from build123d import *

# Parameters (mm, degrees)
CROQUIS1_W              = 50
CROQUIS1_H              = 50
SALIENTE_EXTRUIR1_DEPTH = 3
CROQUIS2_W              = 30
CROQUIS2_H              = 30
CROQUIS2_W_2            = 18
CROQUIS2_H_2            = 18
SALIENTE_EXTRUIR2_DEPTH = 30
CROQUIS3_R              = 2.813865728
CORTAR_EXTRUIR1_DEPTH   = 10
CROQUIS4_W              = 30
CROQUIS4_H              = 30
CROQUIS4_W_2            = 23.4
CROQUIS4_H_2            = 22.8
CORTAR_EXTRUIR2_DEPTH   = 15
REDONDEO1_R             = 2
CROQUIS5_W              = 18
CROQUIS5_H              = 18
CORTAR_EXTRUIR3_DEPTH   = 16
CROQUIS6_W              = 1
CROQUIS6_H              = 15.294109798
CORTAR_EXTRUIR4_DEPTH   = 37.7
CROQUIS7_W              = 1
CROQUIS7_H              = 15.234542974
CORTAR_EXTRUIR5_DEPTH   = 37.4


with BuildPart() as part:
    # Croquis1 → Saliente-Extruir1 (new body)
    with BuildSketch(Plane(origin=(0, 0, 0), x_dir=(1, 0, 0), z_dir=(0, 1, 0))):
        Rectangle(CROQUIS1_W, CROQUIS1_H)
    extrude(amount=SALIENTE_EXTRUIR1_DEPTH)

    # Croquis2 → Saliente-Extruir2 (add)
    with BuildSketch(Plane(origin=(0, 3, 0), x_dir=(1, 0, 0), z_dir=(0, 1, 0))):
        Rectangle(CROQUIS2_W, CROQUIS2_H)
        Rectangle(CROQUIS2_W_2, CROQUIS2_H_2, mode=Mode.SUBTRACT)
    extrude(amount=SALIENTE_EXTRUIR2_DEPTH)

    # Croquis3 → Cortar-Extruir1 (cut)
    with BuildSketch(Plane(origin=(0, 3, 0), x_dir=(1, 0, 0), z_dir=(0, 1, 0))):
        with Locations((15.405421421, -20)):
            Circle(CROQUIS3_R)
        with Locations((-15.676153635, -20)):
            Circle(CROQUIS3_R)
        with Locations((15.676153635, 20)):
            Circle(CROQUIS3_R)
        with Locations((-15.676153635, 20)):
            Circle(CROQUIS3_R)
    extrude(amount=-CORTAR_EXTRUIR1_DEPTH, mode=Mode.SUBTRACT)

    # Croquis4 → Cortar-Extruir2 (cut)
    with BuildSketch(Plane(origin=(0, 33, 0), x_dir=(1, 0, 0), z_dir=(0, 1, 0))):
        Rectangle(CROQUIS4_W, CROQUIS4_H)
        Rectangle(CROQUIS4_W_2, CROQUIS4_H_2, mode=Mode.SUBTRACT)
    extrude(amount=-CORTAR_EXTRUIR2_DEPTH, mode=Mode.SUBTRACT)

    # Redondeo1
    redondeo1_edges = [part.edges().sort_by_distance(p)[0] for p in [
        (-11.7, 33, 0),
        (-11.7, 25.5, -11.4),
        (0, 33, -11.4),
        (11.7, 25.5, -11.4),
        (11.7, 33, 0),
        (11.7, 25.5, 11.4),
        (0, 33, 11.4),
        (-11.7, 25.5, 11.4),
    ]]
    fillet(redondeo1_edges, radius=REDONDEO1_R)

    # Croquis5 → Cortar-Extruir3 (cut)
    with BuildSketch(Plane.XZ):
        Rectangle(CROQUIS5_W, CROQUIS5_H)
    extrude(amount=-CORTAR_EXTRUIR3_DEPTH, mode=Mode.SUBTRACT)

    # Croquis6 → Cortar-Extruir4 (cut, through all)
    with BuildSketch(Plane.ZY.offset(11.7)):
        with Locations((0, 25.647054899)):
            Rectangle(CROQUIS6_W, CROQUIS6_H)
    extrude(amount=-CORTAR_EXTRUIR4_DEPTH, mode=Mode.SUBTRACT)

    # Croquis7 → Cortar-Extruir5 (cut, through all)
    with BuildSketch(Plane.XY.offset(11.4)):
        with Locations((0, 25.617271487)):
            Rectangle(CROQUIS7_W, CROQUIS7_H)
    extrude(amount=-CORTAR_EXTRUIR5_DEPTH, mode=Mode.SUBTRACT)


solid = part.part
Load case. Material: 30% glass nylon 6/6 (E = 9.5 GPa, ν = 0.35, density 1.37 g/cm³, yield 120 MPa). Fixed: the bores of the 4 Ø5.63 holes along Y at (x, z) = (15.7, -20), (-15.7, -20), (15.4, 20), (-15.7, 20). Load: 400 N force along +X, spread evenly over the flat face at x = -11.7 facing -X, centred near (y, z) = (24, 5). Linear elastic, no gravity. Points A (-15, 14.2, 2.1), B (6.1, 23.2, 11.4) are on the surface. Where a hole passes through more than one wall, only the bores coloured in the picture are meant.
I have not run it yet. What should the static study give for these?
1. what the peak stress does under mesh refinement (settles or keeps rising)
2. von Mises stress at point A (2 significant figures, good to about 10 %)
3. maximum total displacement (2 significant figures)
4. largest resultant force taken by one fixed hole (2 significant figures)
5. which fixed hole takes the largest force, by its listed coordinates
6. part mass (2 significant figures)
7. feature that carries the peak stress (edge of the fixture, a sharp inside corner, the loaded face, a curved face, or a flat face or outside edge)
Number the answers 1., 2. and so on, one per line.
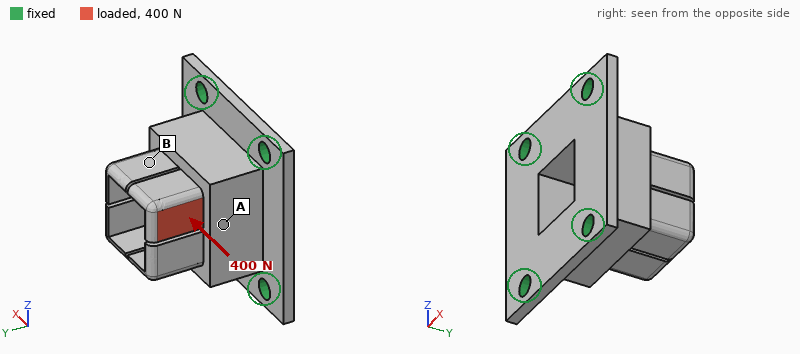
1. keeps rising
2. 16 MPa
3. 0.48 mm
4. 280 N
5. (15.4, 20)
6. 24 g
7. a sharp inside corner
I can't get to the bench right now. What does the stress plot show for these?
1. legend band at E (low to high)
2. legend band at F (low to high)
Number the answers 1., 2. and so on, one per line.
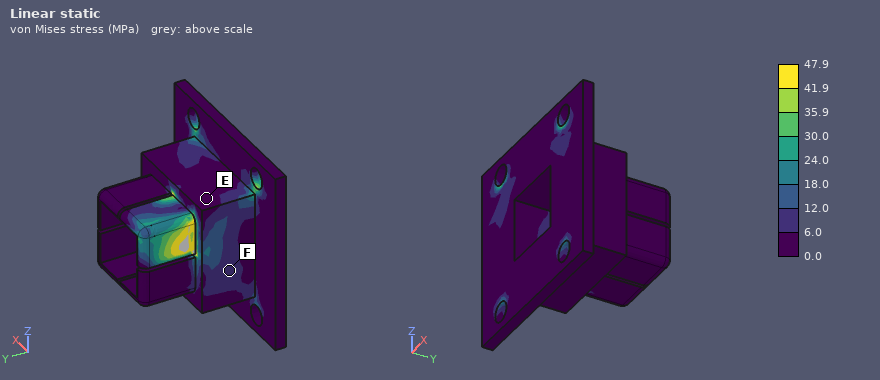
1. 0.0 to 6.0 MPa
2. 6.0 to 12.0 MPa
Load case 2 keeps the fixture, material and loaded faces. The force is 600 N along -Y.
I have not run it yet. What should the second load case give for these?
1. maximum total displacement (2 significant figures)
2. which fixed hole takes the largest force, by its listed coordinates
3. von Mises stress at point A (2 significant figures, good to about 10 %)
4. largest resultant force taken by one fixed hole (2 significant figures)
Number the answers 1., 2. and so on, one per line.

1. 0.17 mm
2. (-15.7, 20)
3. 2.9 MPa
4. 360 N
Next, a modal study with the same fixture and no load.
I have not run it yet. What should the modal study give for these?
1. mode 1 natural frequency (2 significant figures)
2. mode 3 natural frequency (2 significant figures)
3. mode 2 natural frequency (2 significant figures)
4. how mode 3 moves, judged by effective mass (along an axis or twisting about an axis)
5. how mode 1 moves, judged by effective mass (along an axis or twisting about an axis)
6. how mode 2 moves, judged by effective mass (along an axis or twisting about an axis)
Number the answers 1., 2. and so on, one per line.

1. 4800 Hz
2. 6200 Hz
3. 5600 Hz
4. along Y
5. along X
6. along Z
